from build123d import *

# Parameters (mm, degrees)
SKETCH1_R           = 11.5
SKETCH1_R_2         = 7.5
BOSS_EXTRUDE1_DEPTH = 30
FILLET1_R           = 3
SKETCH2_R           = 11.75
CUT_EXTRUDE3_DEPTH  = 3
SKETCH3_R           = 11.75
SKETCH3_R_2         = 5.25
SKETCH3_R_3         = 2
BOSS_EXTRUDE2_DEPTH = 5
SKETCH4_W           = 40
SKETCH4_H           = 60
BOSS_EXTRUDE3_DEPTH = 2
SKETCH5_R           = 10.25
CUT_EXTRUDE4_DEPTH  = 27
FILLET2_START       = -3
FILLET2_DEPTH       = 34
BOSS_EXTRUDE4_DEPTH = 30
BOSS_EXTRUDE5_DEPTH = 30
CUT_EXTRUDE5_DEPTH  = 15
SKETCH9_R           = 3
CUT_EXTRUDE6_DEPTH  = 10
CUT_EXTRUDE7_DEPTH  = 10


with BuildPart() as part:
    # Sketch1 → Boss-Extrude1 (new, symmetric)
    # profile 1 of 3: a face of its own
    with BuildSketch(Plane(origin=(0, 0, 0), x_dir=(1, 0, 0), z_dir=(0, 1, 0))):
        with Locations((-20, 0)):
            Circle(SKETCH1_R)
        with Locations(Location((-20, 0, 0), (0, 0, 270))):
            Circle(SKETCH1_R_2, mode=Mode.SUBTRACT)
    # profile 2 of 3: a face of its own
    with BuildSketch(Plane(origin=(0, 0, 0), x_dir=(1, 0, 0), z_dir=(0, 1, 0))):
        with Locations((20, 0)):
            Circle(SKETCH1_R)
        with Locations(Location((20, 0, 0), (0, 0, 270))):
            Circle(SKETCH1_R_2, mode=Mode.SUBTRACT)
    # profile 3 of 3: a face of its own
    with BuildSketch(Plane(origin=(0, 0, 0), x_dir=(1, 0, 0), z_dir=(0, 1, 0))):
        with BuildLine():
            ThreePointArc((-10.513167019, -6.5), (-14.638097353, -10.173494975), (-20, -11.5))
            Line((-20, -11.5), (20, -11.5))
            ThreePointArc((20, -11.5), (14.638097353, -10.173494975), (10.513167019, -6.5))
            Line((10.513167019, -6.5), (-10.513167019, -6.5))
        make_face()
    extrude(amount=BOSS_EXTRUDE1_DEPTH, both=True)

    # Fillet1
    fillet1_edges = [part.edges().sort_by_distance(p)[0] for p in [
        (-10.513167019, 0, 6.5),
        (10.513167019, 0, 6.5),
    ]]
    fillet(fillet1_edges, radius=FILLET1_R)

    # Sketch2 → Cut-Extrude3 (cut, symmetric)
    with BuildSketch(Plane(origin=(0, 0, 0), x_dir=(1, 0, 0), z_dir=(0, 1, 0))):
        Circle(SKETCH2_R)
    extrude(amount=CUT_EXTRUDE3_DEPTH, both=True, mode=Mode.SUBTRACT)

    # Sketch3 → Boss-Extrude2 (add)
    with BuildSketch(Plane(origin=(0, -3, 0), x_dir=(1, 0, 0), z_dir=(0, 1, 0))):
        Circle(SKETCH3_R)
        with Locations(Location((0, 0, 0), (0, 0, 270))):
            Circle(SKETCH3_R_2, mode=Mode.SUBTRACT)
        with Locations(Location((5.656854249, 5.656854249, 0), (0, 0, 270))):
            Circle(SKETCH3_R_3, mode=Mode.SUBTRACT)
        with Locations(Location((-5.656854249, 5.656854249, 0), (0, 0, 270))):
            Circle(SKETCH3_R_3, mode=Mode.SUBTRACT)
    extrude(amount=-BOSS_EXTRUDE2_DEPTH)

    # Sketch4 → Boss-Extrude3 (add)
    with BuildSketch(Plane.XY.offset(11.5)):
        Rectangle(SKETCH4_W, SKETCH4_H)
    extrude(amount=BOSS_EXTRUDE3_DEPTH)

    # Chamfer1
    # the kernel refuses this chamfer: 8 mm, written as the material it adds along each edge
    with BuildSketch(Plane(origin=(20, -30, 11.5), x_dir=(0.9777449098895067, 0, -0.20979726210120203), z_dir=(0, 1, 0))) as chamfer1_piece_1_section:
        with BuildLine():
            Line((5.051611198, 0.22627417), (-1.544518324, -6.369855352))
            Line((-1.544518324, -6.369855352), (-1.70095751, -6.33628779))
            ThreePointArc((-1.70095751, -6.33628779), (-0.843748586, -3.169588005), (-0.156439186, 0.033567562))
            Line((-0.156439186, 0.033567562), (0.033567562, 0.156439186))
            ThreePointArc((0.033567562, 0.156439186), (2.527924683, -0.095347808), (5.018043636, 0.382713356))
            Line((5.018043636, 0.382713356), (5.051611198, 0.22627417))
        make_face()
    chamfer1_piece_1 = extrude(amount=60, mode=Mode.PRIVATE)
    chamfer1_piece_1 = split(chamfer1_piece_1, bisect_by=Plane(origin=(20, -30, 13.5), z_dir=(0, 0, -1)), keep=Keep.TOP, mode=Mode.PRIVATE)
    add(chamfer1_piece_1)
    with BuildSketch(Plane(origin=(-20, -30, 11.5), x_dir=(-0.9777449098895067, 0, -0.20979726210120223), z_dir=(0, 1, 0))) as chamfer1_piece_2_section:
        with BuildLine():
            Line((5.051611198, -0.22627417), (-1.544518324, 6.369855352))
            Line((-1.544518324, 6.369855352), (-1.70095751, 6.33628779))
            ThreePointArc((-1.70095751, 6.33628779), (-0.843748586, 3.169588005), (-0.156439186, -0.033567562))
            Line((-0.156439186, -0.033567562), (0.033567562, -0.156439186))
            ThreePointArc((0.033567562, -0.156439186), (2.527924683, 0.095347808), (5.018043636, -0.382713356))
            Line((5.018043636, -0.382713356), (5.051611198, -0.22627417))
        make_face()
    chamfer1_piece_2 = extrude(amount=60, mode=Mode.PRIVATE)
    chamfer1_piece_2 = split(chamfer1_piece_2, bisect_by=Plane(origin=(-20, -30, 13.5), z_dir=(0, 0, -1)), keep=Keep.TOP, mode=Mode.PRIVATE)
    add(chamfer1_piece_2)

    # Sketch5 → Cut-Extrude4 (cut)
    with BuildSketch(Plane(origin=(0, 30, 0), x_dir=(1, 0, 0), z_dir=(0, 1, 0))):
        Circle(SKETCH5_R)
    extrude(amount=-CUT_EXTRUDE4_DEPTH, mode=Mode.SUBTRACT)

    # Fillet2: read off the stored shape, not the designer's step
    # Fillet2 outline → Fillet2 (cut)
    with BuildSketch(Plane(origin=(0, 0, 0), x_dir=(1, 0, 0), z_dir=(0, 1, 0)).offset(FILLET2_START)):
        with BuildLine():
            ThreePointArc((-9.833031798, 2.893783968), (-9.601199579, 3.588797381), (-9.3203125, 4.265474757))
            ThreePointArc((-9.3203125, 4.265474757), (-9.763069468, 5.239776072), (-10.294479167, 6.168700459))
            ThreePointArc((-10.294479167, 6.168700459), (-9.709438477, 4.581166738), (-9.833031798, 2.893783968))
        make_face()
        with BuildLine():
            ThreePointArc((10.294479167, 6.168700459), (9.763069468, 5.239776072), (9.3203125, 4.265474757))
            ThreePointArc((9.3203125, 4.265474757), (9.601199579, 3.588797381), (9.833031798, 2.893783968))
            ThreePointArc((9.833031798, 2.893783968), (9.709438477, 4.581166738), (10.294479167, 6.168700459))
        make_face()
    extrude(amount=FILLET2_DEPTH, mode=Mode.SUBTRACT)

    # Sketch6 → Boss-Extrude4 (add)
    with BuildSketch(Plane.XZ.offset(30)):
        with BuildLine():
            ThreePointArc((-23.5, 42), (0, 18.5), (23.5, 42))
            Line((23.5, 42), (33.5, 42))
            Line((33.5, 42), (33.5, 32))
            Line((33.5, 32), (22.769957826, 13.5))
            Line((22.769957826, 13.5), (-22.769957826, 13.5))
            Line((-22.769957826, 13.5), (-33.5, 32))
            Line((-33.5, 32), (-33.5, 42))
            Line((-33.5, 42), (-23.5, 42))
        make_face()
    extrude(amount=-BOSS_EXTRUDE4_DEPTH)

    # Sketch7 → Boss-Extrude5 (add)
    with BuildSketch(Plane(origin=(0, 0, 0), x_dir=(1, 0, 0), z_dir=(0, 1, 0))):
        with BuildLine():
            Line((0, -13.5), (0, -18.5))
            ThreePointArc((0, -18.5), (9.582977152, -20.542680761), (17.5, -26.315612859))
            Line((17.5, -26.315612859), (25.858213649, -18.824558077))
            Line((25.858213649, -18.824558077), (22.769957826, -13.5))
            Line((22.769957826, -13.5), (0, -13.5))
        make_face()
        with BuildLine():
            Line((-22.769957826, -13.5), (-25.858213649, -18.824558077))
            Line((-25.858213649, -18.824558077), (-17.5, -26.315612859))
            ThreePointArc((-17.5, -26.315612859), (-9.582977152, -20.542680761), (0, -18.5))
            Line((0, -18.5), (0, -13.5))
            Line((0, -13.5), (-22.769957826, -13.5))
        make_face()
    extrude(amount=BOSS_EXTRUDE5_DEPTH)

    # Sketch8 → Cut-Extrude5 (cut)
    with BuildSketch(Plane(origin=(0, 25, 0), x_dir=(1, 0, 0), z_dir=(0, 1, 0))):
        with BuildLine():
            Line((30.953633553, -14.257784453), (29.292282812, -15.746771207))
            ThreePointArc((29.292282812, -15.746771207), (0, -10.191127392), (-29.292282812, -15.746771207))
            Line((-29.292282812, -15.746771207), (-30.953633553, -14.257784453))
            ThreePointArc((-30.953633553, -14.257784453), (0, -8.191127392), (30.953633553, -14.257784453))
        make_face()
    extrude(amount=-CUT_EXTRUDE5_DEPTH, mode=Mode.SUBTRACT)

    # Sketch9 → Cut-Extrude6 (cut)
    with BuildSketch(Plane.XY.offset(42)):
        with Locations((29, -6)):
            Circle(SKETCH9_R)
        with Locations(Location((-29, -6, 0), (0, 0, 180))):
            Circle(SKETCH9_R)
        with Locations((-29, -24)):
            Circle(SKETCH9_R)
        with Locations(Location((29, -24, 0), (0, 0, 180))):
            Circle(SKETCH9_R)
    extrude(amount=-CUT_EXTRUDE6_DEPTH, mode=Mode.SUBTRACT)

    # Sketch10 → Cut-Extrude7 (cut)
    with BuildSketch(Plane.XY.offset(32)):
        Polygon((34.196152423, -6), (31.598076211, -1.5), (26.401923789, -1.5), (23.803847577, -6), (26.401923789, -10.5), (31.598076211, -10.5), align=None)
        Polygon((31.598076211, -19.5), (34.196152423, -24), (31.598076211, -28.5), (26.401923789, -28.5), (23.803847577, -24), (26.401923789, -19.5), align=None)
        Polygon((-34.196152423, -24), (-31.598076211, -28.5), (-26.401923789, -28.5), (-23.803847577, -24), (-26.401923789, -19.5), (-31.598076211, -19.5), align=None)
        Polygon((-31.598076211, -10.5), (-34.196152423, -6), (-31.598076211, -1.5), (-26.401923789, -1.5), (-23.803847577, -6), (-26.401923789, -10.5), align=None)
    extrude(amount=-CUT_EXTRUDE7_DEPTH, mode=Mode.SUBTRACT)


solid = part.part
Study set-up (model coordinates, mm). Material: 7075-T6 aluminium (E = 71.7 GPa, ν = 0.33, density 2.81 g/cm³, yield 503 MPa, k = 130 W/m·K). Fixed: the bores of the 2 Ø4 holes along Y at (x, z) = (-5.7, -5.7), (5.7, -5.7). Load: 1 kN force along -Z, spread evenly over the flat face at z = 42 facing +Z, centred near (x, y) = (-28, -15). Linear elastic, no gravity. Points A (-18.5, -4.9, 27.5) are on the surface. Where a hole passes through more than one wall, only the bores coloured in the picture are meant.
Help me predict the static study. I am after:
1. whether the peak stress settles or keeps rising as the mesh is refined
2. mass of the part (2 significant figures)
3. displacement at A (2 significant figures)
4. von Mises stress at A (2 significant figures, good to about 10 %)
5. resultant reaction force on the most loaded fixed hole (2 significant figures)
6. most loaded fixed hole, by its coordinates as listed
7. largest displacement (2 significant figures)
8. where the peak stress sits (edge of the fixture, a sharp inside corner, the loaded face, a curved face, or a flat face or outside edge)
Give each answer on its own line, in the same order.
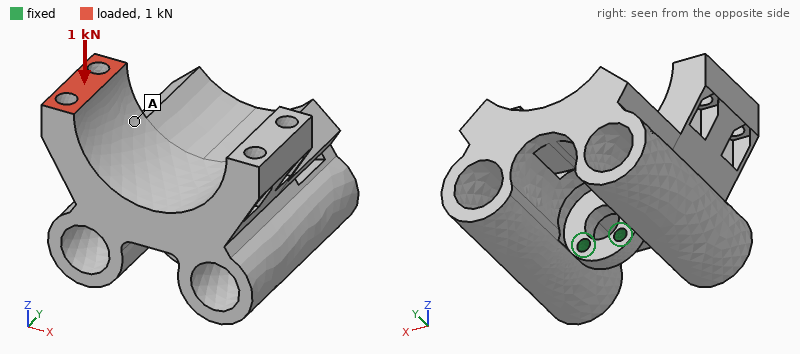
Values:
keeps rising
210 g
0.12 mm
11 MPa
2.2 kN
(-5.7, -5.7)
0.23 mm
a sharp inside corner
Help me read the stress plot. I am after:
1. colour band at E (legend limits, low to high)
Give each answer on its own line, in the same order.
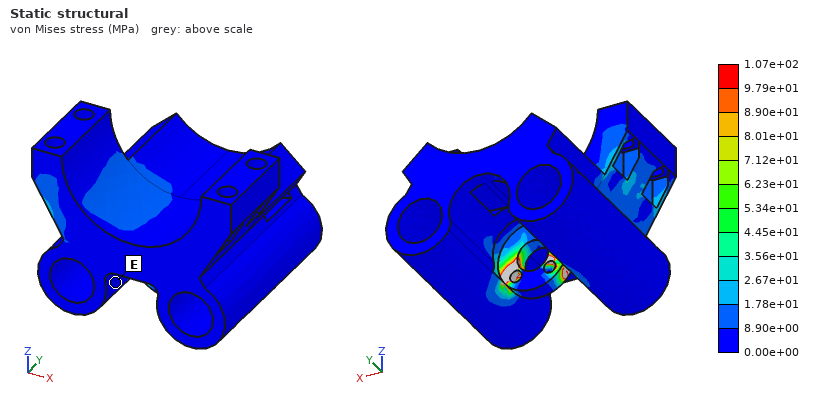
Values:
0.00e+00 to 8.90e+00 MPa
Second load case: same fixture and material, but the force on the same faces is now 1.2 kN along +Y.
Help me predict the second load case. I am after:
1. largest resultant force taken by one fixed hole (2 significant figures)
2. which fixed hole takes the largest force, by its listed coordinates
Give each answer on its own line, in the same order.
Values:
2.3 kN
(-5.7, -5.7)
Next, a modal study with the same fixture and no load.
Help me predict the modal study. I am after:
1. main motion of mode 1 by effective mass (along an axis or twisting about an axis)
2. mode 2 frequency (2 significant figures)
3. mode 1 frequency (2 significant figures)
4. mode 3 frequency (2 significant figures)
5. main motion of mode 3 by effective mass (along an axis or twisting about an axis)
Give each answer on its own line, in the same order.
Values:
along Y
1600 Hz
690 Hz
1800 Hz
along X
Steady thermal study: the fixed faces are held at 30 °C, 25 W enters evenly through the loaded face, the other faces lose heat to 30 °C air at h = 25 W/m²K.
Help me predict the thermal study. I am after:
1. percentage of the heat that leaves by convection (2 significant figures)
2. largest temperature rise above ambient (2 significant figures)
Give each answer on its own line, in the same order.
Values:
33 %
36 K
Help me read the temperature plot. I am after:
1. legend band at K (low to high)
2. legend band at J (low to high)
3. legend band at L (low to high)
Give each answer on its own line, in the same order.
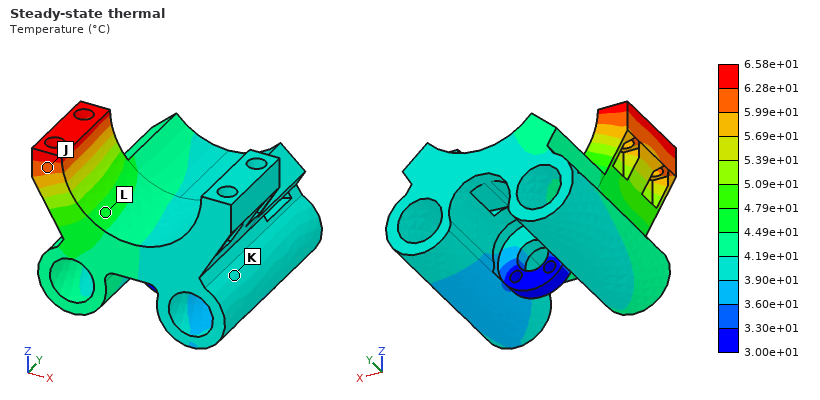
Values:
3.90e+01 to 4.19e+01 °C
5.99e+01 to 6.28e+01 °C
4.49e+01 to 4.79e+01 °C
